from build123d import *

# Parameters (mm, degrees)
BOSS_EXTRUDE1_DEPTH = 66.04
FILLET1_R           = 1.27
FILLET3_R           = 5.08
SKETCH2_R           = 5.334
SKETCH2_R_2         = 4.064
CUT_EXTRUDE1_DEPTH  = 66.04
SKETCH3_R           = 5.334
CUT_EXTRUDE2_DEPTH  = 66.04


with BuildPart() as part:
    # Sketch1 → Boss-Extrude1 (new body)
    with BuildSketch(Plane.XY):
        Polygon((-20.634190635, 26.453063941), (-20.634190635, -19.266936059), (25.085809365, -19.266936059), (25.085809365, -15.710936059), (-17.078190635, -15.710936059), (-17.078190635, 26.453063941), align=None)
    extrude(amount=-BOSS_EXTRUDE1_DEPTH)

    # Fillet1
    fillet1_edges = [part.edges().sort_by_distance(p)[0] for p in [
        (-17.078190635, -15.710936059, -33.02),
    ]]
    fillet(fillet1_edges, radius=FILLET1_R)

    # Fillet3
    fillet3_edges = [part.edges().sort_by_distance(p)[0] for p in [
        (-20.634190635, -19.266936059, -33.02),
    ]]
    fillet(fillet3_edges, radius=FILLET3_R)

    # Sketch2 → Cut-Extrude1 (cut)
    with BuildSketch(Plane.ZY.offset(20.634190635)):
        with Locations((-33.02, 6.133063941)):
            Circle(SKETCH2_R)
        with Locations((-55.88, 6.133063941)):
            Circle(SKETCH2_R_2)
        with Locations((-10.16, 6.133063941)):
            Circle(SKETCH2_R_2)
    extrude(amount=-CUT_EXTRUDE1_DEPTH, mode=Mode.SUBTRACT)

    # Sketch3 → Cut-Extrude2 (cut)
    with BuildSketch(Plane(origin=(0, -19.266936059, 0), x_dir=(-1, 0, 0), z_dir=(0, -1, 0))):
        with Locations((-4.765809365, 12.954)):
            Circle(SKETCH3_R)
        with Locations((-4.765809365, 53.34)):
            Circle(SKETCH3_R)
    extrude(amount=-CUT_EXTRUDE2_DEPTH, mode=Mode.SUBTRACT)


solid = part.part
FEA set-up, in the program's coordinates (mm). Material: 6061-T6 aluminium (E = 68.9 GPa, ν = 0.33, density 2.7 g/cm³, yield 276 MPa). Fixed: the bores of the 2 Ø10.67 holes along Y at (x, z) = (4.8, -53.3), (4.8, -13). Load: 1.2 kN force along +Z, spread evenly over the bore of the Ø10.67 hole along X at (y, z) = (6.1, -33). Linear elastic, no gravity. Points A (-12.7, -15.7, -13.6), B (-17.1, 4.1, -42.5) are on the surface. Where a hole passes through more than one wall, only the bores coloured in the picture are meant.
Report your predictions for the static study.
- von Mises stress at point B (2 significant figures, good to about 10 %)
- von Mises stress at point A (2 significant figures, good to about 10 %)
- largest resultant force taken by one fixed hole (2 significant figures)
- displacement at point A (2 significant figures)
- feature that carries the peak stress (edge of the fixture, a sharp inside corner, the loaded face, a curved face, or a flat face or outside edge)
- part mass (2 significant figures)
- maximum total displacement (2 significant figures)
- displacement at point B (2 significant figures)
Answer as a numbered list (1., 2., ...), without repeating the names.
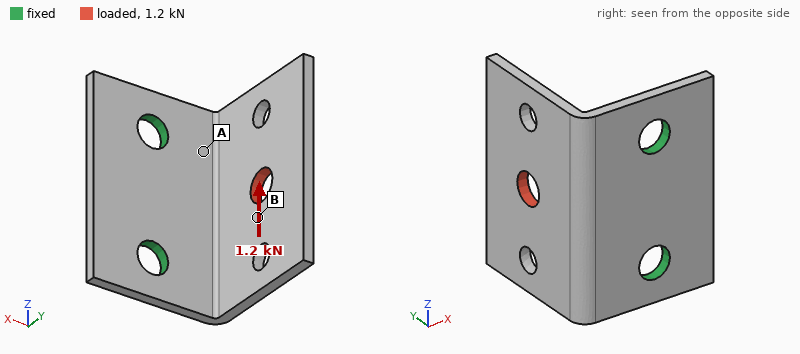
1. 29 MPa
2. 61 MPa
3. 1.0 kN
4. 0.067 mm
5. a flat face or outside edge
6. 51 g
7. 0.36 mm
8. 0.15 mm
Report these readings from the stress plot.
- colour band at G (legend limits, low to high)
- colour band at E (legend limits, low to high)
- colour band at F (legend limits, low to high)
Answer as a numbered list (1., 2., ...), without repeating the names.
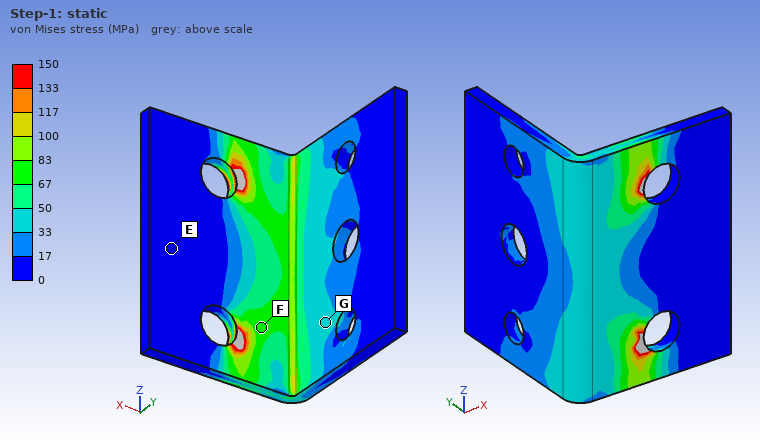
1. 33 to 50 MPa
2. 0 to 17 MPa
3. 67 to 83 MPa
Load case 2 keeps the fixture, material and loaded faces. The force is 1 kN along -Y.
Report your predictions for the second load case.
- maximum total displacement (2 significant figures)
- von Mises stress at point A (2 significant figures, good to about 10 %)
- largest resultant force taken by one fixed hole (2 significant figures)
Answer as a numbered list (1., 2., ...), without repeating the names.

1. 0.54 mm
2. 38 MPa
3. 500 N
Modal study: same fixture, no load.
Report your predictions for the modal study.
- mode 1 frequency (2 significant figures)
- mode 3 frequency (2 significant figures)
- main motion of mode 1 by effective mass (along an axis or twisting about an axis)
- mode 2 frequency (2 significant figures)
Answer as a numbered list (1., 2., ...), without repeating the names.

1. 910 Hz
2. 2900 Hz
3. along X
4. 1800 Hz
